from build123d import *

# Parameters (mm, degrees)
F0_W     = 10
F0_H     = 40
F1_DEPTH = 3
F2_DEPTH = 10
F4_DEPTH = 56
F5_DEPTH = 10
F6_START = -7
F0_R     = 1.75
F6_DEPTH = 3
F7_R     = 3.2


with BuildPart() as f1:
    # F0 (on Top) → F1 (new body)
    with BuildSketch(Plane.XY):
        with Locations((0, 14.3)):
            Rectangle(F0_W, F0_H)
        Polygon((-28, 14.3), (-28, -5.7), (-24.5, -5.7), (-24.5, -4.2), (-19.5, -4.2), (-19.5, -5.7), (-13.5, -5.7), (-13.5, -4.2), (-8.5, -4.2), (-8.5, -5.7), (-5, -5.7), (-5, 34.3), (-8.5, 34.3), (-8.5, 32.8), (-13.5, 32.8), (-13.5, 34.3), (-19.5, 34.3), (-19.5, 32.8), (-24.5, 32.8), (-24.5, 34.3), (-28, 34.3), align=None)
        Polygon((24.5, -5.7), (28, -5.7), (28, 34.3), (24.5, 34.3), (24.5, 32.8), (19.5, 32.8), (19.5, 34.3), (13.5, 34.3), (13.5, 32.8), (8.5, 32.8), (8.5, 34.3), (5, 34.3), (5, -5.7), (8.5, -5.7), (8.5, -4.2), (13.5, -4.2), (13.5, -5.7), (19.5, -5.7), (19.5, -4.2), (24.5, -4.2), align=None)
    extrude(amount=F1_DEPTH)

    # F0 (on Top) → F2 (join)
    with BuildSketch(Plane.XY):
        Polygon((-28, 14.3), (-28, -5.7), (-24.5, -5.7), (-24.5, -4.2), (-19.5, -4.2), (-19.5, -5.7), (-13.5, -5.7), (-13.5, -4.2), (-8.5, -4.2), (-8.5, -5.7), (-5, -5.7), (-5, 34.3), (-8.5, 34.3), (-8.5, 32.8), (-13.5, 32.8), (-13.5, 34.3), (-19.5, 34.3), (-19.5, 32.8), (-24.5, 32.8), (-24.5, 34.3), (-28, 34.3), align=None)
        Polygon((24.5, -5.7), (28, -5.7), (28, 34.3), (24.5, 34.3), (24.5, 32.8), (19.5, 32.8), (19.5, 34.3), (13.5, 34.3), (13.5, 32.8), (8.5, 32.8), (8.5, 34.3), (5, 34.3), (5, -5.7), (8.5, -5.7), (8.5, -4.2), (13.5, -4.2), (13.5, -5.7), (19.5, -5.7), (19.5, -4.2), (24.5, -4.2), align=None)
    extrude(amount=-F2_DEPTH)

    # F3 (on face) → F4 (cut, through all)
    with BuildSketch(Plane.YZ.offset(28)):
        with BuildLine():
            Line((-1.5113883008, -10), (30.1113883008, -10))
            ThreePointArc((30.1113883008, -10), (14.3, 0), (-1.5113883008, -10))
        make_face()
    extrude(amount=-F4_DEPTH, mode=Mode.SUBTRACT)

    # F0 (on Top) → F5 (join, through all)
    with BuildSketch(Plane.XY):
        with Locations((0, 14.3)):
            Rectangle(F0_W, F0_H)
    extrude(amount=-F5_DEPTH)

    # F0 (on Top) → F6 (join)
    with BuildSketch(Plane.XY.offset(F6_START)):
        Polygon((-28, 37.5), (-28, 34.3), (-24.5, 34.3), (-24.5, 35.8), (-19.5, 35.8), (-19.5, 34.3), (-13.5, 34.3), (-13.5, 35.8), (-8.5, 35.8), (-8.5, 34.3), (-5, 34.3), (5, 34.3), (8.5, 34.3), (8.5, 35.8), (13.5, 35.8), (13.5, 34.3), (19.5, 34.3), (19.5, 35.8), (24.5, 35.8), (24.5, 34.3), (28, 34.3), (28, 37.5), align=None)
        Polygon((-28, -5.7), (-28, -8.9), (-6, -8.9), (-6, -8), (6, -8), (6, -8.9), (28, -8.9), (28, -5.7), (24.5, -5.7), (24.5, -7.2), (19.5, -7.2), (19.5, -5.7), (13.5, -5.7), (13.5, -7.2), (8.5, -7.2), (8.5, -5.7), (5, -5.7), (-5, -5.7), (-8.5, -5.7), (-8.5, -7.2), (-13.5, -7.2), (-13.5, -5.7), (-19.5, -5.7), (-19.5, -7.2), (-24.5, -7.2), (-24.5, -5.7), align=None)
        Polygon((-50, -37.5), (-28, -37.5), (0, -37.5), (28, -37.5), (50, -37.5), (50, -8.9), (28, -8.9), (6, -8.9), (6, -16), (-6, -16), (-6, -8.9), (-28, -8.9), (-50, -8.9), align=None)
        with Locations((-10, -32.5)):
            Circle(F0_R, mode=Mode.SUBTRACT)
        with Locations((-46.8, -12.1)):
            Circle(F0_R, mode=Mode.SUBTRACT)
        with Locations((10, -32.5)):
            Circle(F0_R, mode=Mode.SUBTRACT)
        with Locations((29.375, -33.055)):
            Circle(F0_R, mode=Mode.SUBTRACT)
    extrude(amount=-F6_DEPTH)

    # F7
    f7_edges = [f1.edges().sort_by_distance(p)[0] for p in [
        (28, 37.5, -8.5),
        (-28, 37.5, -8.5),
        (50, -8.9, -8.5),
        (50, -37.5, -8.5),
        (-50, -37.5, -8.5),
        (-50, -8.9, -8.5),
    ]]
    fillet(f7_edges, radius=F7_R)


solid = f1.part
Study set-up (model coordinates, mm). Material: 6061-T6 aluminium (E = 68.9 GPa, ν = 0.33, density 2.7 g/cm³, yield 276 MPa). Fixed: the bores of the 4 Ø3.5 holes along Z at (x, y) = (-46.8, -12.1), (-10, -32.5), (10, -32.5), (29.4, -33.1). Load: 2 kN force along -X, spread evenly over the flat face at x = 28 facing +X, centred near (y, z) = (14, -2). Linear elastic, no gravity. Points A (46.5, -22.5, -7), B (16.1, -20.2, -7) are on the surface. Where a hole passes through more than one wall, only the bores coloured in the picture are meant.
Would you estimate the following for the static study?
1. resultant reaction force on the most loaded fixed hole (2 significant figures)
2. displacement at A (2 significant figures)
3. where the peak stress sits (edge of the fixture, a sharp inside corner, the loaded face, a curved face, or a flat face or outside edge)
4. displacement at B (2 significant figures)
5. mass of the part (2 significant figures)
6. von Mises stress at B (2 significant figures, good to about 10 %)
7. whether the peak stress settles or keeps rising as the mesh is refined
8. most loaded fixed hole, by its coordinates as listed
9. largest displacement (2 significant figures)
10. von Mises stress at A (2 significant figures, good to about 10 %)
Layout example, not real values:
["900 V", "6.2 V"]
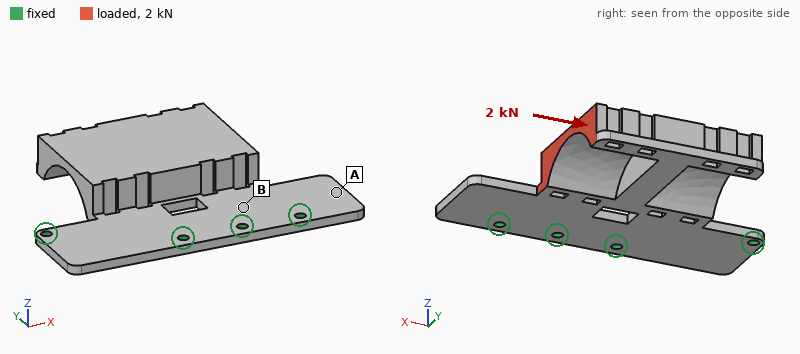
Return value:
["1.5 kN", "0.044 mm", "edge of the fixture", "0.041 mm", "73 g", "41 MPa", "keeps rising", "(29.4, -33.1)", "0.24 mm", "19 MPa"]
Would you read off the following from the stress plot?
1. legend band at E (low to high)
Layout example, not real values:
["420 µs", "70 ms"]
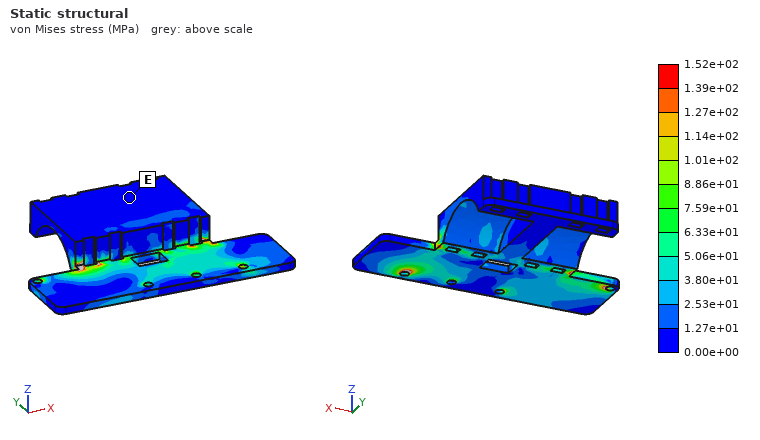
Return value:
["0.00e+00 to 1.27e+01 MPa"]
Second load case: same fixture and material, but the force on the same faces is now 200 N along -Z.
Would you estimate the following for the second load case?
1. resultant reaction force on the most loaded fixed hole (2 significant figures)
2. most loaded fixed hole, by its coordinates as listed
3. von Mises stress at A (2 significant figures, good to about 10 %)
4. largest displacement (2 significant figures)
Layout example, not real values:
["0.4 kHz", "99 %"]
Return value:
["140 N", "(29.4, -33.1)", "32 MPa", "1.1 mm"]
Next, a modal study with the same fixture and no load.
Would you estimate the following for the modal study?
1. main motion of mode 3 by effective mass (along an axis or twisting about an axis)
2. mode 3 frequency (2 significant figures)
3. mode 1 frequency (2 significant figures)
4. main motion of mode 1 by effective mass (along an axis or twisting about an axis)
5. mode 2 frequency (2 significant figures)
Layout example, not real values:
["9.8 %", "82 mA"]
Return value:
["along Z", "3000 Hz", "380 Hz", "along Z", "1900 Hz"]
